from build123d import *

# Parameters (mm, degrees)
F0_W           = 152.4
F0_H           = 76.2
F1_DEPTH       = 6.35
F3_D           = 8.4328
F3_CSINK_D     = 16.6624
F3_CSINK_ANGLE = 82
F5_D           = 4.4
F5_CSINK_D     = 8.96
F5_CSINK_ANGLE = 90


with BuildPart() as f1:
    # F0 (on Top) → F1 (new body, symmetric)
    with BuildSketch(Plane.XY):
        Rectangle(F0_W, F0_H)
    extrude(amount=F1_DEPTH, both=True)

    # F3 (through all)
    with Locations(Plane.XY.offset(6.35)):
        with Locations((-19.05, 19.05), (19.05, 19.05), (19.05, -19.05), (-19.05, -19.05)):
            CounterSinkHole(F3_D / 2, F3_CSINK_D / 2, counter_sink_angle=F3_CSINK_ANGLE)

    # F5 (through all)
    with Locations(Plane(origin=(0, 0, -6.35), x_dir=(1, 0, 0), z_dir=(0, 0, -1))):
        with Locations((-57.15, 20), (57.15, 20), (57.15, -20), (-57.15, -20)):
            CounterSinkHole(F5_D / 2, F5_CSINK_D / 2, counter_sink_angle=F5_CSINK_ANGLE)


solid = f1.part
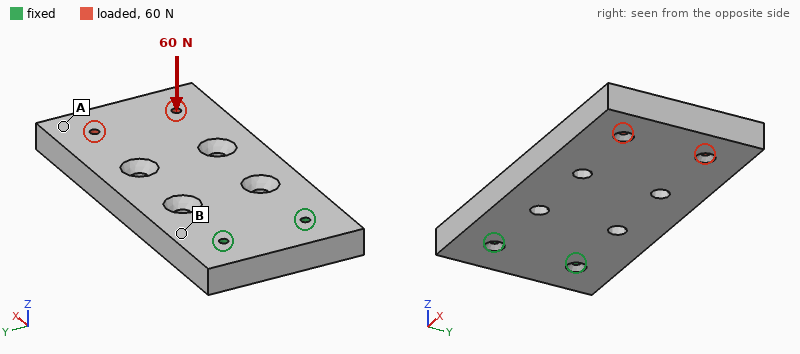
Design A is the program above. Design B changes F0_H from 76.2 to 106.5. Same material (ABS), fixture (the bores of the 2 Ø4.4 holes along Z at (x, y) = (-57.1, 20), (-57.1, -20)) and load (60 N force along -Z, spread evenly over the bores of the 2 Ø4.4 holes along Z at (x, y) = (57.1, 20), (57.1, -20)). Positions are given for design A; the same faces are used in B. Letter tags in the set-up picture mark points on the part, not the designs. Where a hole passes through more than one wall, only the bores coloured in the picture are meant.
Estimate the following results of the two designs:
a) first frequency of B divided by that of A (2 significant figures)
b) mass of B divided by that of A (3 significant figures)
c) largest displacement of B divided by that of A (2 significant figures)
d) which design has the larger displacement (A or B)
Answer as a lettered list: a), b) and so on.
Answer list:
a) 0.95
b) 1.41
c) 0.78
d) A
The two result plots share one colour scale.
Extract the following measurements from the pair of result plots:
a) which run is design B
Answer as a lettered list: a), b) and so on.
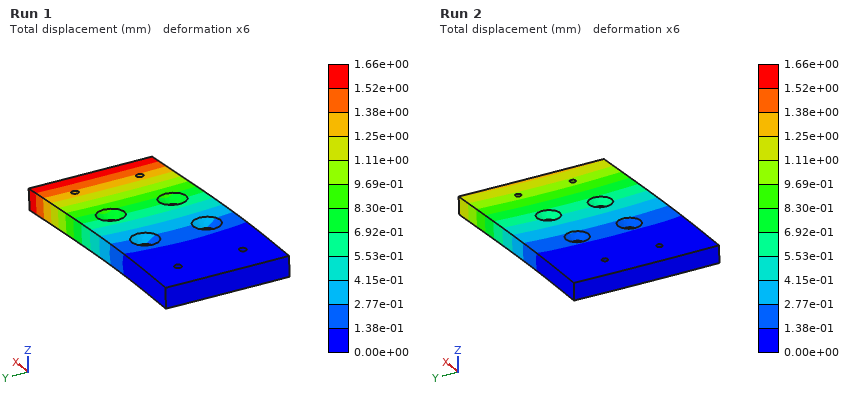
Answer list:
a) Run 2
